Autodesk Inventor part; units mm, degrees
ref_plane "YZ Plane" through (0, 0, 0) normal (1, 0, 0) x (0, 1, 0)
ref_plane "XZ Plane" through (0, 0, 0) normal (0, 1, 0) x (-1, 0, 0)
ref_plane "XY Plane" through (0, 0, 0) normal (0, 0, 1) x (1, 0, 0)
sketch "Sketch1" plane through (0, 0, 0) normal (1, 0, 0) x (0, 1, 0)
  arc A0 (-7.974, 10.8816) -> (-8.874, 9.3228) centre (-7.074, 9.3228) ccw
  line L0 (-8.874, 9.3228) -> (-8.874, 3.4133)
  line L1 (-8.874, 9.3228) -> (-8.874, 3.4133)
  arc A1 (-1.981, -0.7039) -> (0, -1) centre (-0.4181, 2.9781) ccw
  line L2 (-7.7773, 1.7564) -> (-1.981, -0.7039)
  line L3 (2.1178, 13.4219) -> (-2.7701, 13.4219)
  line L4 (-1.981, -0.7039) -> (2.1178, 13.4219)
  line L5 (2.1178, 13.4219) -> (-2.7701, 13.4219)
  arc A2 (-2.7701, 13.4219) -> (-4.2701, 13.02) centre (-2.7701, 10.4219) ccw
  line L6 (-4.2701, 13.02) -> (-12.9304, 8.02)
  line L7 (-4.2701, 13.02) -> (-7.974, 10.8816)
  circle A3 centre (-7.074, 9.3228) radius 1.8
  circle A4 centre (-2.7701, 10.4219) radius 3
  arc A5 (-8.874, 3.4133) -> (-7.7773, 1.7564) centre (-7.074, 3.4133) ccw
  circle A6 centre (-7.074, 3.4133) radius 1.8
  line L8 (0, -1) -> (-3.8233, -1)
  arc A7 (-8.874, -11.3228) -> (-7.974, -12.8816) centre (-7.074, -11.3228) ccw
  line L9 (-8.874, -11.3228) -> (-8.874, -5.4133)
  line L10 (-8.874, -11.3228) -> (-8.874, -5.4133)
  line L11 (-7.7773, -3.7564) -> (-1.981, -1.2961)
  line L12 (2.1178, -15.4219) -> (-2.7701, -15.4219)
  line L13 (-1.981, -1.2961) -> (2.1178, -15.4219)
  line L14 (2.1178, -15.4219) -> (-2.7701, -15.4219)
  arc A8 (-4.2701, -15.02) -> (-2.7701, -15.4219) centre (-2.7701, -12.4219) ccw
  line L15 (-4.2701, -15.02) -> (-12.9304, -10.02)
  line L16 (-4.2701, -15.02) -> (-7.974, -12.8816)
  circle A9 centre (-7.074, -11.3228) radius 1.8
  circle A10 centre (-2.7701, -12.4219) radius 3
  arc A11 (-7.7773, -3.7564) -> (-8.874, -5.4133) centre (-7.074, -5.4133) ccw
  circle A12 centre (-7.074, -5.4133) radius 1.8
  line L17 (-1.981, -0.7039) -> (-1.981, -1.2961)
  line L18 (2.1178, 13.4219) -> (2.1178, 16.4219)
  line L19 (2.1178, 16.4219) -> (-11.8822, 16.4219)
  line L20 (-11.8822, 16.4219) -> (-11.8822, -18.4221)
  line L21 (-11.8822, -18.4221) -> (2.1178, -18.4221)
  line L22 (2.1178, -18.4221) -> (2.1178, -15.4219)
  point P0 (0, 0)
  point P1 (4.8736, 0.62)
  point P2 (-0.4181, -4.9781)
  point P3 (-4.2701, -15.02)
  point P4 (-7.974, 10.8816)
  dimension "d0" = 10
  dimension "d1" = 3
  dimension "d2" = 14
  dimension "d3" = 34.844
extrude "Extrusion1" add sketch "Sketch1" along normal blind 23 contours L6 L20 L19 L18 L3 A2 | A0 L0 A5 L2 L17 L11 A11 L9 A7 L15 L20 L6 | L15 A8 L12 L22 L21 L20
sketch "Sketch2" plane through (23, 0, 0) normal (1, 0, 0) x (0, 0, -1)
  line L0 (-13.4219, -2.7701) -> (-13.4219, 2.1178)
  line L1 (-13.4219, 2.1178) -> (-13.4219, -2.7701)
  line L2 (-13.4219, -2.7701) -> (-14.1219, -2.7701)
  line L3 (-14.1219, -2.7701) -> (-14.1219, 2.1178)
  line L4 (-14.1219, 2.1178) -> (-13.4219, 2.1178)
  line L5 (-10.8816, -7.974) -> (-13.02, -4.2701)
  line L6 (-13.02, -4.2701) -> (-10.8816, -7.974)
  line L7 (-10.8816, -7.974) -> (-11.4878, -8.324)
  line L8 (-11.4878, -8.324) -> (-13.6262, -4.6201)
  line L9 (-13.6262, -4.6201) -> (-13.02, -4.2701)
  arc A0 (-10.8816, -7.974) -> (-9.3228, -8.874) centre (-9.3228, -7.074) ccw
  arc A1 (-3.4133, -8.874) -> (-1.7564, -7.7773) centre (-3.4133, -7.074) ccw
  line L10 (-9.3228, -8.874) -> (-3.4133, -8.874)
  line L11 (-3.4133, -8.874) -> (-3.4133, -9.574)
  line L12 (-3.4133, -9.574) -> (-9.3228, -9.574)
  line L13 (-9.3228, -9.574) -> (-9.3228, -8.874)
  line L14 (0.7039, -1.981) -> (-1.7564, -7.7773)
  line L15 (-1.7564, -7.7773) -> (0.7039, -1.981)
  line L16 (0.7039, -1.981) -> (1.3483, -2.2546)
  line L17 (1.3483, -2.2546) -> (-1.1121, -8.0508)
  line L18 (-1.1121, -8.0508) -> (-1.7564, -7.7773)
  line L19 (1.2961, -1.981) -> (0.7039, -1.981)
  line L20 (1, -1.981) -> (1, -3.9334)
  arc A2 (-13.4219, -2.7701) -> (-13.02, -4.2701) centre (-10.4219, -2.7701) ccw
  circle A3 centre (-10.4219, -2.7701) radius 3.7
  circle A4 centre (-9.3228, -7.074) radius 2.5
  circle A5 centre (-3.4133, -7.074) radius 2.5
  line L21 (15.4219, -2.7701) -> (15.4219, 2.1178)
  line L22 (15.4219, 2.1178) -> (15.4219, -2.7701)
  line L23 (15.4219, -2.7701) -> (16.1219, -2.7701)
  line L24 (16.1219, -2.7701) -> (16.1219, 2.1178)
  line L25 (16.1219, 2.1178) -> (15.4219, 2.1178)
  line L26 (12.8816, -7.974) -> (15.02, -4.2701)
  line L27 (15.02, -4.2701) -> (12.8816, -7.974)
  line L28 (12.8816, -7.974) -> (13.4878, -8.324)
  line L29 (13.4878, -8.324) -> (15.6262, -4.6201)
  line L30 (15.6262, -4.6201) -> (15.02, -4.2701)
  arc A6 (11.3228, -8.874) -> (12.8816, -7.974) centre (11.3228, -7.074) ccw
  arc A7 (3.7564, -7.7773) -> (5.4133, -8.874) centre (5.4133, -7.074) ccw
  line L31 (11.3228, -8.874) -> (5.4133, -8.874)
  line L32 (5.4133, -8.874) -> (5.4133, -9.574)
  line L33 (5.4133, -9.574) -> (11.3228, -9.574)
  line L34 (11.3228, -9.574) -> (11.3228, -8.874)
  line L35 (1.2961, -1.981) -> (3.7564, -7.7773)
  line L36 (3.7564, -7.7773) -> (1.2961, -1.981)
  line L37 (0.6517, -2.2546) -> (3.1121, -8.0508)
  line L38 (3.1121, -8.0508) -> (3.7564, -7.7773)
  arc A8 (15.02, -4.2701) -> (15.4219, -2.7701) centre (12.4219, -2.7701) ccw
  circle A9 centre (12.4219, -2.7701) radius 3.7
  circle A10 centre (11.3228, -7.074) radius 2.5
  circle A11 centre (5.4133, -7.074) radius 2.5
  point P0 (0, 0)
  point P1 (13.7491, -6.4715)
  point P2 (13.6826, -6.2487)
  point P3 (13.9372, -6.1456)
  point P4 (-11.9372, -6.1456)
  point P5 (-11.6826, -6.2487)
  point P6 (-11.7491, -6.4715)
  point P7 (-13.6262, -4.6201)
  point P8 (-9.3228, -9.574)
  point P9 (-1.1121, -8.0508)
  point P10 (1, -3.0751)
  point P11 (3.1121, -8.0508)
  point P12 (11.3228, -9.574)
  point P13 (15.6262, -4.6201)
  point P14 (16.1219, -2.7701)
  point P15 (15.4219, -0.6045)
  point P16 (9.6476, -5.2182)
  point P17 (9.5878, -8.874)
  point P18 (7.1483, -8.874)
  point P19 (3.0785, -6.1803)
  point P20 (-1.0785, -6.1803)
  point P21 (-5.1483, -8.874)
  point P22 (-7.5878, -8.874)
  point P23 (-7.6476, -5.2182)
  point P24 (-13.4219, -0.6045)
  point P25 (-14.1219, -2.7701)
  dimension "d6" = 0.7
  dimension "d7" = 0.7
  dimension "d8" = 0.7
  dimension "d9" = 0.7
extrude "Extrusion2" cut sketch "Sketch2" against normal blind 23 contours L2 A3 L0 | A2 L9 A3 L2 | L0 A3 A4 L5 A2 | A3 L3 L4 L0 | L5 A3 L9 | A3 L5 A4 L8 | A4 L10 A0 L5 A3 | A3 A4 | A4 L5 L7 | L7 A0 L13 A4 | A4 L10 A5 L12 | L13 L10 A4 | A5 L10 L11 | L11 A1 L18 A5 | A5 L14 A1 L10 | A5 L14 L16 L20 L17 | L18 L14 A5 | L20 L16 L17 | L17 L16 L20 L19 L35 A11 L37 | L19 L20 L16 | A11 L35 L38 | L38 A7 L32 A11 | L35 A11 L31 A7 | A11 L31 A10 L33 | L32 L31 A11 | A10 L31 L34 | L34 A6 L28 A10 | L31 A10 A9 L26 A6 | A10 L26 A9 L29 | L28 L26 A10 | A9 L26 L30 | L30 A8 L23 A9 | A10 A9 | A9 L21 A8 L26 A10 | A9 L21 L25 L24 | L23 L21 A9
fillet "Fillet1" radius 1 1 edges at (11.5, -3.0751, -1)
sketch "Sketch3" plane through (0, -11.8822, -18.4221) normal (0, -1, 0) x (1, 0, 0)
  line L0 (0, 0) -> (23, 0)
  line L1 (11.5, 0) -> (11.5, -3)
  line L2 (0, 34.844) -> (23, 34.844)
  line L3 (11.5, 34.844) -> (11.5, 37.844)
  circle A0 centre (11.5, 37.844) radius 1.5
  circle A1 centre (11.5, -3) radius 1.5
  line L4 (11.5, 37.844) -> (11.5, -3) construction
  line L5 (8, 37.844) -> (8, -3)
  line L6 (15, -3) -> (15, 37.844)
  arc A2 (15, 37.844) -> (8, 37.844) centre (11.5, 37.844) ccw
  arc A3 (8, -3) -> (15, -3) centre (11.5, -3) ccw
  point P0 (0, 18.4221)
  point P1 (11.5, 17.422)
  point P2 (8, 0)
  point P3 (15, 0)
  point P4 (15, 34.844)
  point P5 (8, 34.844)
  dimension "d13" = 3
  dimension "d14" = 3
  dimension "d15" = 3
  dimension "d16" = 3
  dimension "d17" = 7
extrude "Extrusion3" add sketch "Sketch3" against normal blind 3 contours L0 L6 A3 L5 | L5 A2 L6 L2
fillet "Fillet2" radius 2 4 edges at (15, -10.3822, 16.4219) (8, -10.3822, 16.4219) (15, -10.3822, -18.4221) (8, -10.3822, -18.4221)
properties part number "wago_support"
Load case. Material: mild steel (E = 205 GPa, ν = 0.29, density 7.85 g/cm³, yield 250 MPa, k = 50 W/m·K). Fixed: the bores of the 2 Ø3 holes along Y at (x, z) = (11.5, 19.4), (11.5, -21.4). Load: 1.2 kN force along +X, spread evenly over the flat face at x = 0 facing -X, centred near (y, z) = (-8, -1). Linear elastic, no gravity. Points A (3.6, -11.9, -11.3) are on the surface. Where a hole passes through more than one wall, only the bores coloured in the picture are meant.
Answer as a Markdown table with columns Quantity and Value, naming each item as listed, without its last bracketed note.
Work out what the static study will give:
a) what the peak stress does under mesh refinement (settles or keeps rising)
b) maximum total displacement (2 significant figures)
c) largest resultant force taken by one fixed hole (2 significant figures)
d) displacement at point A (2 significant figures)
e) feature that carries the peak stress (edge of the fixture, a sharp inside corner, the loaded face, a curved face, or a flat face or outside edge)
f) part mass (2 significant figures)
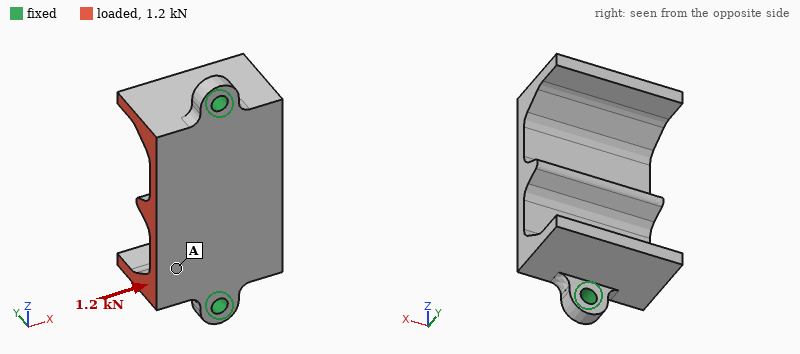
| Quantity | Value |
|---|---|
| what the peak stress does under mesh refinement | keeps rising |
| maximum total displacement | 17 µm |
| largest resultant force taken by one fixed hole | 600 N |
| displacement at point A | 7.1 µm |
| feature that carries the peak stress | edge of the fixture |
| part mass | 33 g |
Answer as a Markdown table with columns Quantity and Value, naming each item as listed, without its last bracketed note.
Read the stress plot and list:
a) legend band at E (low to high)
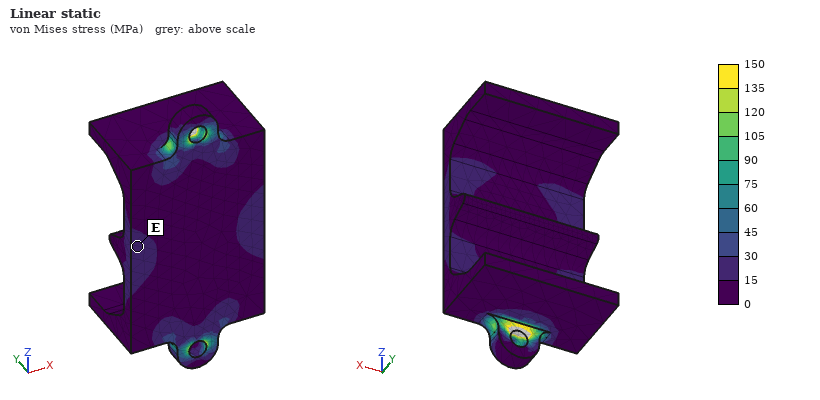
| Quantity | Value |
|---|---|
| legend band at E | 15 to 30 MPa |
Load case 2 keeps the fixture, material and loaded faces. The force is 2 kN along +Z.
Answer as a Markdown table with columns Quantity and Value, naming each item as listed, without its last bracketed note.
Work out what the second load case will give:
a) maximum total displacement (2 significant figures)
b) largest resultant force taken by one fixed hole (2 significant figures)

| Quantity | Value |
|---|---|
| maximum total displacement | 29 µm |
| largest resultant force taken by one fixed hole | 1.2 kN |
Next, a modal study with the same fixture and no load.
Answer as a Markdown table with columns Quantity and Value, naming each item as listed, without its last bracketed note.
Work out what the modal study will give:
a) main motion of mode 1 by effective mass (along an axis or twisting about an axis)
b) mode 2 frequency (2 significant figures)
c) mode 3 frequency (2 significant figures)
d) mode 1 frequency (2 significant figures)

| Quantity | Value |
|---|---|
| main motion of mode 1 by effective mass | along Y |
| mode 2 frequency | 6200 Hz |
| mode 3 frequency | 10 kHz |
| mode 1 frequency | 5800 Hz |
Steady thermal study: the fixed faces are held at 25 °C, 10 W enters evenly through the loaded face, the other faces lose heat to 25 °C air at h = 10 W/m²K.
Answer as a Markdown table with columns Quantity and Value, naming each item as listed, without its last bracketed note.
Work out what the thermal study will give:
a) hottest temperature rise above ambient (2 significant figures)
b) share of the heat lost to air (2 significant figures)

| Quantity | Value |
|---|---|
| hottest temperature rise above ambient | 34 K |
| share of the heat lost to air | 6.1 % |
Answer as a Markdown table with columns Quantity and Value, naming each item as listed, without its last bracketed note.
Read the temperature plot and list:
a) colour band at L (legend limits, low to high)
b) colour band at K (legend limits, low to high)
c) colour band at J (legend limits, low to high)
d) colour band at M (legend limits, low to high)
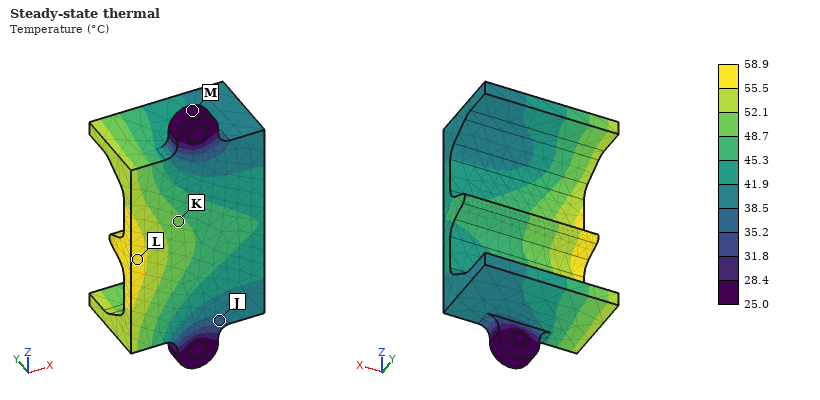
| Quantity | Value |
|---|---|
| colour band at L | 55.5 to 58.9 °C |
| colour band at K | 48.7 to 52.1 °C |
| colour band at J | 35.2 to 38.5 °C |
| colour band at M | 25.0 to 28.4 °C |
